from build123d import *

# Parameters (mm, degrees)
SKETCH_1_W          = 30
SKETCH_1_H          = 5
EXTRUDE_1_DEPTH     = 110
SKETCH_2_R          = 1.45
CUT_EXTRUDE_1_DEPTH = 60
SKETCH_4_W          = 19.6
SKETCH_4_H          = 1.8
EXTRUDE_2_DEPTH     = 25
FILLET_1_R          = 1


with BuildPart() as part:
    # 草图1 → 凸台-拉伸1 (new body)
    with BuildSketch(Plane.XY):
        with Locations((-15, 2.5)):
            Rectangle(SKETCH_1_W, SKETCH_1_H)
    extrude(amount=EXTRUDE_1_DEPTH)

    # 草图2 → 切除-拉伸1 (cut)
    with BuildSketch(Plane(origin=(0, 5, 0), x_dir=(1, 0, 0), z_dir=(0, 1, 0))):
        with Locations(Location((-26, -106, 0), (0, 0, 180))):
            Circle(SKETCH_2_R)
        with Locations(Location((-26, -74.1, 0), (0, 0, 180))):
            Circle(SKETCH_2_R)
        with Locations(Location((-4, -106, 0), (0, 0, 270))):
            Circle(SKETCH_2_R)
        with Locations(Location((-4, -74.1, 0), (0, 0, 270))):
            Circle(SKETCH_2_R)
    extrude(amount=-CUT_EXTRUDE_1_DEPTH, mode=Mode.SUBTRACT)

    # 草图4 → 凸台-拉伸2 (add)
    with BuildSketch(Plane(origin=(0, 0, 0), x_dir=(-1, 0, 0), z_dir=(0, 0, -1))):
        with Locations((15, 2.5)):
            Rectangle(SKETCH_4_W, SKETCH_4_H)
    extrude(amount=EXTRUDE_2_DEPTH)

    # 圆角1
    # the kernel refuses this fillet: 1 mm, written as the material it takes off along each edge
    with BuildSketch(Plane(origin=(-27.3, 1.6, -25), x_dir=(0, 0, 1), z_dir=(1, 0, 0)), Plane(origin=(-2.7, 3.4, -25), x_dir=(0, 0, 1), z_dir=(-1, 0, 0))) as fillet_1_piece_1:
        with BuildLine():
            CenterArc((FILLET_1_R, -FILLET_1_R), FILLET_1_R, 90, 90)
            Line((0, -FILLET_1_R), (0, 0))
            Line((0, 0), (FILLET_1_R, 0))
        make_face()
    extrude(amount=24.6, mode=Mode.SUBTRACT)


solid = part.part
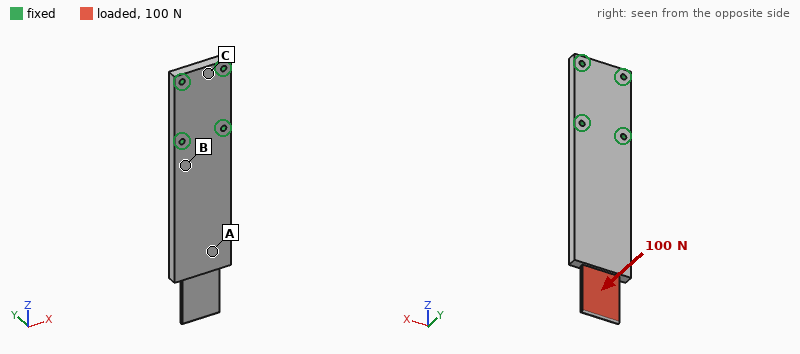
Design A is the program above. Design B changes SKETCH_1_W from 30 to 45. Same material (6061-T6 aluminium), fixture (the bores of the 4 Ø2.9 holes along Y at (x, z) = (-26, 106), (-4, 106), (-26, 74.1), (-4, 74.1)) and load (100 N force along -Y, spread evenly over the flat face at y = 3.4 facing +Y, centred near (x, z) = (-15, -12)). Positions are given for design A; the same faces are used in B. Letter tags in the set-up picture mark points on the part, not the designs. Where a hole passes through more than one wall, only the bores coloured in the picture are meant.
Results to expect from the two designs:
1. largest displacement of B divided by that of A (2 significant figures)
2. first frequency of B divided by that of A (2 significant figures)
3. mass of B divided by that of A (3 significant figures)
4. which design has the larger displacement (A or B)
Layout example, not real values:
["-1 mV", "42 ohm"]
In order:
["0.74", "1.1", "1.48", "A"]
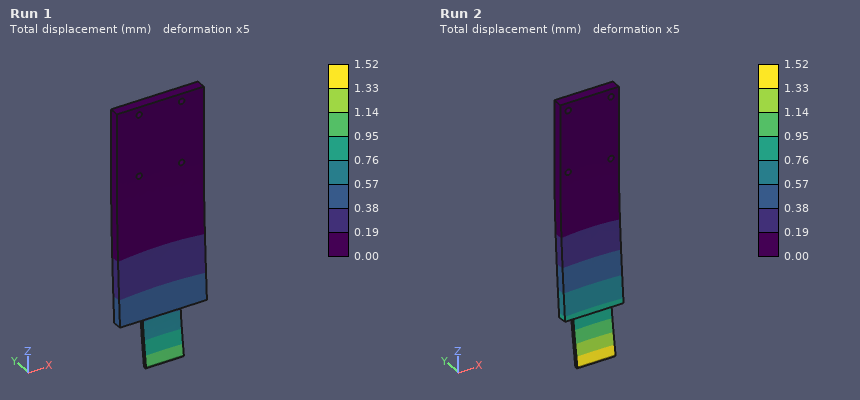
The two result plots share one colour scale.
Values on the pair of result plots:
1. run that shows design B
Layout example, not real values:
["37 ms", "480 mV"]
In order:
["Run 1"]
